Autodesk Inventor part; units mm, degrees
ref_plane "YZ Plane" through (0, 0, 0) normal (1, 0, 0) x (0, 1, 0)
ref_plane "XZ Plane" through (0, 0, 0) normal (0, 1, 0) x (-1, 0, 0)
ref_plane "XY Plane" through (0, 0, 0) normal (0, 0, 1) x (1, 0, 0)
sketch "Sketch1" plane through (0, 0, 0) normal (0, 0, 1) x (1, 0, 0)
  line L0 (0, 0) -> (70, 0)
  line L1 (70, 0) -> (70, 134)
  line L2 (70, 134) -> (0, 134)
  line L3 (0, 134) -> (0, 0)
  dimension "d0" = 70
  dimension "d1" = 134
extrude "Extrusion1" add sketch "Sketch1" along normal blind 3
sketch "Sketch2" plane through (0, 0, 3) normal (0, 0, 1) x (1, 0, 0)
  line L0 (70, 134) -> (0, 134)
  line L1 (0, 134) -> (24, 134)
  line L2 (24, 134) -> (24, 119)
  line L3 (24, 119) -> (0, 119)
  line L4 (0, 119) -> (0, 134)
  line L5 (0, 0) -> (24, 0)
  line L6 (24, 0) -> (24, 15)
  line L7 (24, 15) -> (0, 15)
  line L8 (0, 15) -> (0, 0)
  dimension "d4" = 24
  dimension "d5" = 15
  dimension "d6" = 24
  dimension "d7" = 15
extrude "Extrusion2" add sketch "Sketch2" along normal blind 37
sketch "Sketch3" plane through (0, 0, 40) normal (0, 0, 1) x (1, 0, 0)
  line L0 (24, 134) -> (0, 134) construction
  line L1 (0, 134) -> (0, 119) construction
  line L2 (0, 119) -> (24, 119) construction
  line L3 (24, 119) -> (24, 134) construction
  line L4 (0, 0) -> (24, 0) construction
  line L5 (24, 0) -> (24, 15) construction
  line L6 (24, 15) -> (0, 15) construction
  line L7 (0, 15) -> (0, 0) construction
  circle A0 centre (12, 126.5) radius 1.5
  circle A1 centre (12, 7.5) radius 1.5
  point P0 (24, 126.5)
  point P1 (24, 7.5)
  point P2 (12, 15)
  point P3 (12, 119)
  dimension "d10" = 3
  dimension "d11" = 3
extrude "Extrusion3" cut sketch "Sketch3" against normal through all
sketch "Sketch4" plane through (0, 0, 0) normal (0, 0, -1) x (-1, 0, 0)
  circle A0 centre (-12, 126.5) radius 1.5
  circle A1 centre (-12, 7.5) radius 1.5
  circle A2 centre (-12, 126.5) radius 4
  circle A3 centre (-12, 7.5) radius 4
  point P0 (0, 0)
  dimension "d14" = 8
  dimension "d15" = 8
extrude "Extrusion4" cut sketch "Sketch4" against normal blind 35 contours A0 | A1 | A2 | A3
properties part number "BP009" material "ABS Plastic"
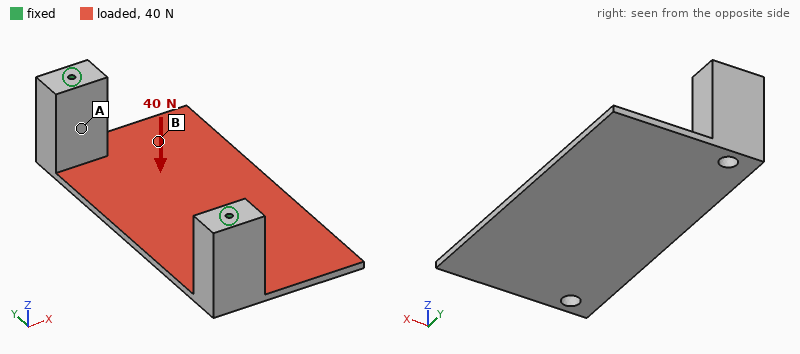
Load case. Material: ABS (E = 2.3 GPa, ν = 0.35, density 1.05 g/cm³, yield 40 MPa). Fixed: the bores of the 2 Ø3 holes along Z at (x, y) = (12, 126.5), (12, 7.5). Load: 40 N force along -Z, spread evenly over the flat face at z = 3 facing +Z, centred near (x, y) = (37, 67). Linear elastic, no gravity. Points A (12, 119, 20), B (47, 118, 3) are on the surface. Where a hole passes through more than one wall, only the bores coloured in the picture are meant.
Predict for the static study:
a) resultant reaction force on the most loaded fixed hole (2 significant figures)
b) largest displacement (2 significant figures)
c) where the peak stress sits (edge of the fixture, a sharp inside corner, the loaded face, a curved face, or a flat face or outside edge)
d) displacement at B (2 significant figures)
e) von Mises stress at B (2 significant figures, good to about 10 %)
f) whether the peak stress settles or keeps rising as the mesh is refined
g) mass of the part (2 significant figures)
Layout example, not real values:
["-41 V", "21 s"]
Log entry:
["23 N", "1.8 mm", "edge of the fixture", "0.59 mm", "1.1 MPa", "keeps rising", "54 g"]
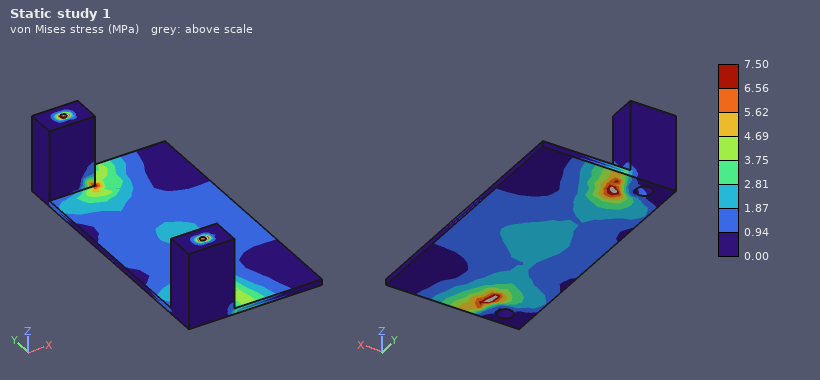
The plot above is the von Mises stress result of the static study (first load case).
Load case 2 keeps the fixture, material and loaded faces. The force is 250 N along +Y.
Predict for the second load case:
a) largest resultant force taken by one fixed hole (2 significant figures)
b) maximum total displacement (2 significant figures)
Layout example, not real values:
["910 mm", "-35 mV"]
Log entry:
["130 N", "1.6 mm"]
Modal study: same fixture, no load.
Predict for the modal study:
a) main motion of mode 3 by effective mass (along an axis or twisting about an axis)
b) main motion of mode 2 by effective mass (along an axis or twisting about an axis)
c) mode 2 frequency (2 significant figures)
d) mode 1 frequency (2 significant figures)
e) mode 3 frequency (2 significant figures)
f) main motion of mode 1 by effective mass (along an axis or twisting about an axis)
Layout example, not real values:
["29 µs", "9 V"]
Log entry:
["along X", "along Y", "330 Hz", "190 Hz", "390 Hz", "along Z"]
